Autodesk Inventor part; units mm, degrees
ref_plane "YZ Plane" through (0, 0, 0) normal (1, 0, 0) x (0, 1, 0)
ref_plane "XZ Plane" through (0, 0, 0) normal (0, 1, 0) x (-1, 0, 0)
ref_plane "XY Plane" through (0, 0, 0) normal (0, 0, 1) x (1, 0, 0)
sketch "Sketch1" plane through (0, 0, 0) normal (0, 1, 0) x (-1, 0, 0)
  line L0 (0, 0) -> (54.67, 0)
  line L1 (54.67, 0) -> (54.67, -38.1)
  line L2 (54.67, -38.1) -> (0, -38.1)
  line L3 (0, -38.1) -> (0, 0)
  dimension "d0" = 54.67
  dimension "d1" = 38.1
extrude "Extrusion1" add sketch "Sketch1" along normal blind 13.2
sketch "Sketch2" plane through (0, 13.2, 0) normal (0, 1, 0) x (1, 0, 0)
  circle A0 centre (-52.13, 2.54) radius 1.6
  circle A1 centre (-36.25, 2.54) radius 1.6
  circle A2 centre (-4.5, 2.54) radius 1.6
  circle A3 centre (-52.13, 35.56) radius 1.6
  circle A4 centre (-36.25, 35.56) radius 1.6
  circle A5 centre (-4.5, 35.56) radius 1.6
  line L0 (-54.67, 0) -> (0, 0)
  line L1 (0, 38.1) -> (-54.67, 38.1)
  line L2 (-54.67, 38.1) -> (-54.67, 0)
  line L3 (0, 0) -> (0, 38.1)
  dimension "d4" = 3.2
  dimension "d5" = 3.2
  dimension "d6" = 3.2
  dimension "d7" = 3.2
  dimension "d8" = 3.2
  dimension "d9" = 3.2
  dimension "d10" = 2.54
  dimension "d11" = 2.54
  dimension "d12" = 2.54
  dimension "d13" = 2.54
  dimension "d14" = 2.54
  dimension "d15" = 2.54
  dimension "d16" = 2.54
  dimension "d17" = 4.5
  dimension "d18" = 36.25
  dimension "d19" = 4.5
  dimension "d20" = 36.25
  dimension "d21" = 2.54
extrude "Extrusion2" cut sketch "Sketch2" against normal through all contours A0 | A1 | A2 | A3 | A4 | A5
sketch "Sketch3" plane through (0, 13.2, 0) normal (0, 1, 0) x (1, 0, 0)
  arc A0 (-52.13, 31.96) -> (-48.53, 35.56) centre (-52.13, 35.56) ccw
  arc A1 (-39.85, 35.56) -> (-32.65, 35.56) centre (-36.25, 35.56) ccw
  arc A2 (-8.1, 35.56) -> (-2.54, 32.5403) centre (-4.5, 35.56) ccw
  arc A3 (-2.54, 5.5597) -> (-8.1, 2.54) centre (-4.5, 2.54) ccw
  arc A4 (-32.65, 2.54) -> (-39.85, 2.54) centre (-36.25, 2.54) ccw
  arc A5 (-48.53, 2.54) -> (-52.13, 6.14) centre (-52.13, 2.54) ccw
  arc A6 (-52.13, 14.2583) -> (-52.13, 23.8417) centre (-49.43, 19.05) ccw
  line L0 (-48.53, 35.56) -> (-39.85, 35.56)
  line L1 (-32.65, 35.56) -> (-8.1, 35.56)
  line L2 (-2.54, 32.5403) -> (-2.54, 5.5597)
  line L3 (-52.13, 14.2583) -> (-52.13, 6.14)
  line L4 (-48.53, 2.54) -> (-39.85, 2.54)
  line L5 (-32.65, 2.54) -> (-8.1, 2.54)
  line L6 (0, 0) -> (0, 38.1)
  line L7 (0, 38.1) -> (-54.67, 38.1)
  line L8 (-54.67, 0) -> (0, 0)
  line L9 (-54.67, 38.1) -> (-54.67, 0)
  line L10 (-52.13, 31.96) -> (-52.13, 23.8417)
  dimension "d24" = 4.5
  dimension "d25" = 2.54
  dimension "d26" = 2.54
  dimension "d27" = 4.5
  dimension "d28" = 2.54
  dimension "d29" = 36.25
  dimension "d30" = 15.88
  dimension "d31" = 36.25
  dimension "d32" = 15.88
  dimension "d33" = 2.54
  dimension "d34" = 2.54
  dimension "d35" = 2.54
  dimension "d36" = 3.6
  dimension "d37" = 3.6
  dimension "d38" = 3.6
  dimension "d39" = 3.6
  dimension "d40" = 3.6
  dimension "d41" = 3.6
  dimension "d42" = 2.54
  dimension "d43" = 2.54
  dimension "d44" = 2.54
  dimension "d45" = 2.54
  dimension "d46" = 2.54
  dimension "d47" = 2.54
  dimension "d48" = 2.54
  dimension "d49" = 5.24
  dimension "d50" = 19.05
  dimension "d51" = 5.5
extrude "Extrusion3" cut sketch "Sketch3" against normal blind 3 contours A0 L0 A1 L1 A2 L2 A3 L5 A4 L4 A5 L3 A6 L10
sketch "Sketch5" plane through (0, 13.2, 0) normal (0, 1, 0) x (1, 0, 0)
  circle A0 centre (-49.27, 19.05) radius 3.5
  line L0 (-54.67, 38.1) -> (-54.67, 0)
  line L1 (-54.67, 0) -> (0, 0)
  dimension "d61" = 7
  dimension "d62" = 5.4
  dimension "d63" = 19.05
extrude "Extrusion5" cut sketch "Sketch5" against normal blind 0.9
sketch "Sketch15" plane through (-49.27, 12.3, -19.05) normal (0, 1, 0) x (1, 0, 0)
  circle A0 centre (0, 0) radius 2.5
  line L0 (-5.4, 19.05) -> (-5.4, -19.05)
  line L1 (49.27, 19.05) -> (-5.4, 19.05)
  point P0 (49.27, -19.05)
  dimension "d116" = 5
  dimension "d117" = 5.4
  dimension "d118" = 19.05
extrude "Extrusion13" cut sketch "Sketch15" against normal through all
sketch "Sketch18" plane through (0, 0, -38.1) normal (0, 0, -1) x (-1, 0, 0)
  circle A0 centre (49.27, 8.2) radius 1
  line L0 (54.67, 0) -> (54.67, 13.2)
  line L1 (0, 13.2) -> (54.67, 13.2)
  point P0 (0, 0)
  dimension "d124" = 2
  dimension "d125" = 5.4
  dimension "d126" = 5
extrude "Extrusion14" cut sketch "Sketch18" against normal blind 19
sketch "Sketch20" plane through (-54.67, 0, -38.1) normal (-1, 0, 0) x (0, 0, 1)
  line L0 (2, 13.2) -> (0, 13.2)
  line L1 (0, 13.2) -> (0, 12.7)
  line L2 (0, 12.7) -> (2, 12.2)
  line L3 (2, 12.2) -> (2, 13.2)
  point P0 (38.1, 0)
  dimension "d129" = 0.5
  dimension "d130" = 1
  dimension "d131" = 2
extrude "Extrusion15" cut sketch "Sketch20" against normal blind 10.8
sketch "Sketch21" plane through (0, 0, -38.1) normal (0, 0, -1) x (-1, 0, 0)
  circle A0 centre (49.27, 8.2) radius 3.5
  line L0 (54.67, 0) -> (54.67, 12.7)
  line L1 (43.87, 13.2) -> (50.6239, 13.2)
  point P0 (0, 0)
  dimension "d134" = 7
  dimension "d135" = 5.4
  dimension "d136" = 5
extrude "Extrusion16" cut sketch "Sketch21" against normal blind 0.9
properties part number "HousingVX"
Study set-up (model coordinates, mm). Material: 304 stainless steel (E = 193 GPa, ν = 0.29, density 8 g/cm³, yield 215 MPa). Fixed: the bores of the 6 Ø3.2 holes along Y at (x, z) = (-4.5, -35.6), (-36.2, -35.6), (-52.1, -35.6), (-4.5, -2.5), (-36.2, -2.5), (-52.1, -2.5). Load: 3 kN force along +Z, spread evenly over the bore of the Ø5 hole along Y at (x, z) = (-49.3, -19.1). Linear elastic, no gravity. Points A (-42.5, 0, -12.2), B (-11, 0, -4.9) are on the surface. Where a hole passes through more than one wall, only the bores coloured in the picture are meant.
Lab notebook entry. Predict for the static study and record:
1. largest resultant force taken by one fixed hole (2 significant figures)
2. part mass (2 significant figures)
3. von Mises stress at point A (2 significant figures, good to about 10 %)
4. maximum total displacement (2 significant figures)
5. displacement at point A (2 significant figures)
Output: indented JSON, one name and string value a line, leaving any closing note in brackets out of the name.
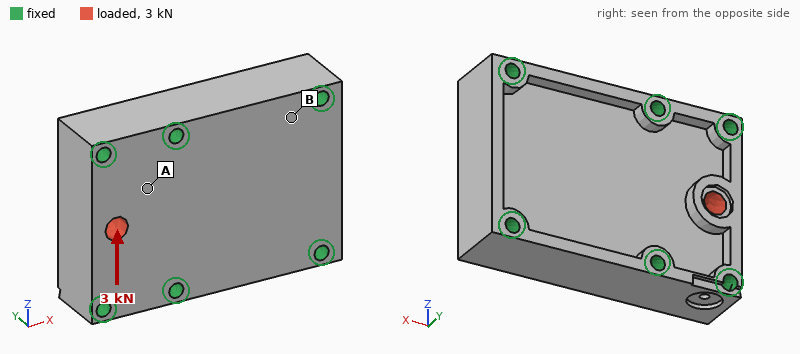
{
  "largest resultant force taken by one fixed hole": "1.0 kN",
  "part mass": "180 g",
  "von Mises stress at point A": "5.3 MPa",
  "maximum total displacement": "1.2 µm",
  "displacement at point A": "0.35 µm"
}
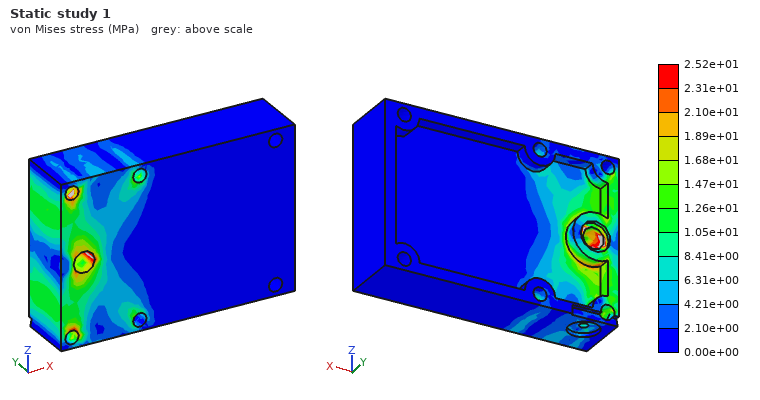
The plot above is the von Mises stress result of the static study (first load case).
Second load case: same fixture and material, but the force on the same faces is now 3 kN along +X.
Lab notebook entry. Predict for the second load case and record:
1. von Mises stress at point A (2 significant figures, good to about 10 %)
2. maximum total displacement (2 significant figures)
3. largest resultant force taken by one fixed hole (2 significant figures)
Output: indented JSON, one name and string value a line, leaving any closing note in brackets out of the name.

{
  "von Mises stress at point A": "11 MPa",
  "maximum total displacement": "2.7 µm",
  "largest resultant force taken by one fixed hole": "910 N"
}
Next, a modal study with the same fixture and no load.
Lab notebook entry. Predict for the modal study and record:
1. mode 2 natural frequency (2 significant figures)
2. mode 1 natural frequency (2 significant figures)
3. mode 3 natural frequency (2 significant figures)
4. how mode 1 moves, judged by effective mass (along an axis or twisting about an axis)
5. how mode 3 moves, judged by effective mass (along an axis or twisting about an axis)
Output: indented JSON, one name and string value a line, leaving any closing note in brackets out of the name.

{
  "mode 2 natural frequency": "33 kHz",
  "mode 1 natural frequency": "24 kHz",
  "mode 3 natural frequency": "37 kHz",
  "how mode 1 moves, judged by effective mass": "along Y",
  "how mode 3 moves, judged by effective mass": "along Z"
}
